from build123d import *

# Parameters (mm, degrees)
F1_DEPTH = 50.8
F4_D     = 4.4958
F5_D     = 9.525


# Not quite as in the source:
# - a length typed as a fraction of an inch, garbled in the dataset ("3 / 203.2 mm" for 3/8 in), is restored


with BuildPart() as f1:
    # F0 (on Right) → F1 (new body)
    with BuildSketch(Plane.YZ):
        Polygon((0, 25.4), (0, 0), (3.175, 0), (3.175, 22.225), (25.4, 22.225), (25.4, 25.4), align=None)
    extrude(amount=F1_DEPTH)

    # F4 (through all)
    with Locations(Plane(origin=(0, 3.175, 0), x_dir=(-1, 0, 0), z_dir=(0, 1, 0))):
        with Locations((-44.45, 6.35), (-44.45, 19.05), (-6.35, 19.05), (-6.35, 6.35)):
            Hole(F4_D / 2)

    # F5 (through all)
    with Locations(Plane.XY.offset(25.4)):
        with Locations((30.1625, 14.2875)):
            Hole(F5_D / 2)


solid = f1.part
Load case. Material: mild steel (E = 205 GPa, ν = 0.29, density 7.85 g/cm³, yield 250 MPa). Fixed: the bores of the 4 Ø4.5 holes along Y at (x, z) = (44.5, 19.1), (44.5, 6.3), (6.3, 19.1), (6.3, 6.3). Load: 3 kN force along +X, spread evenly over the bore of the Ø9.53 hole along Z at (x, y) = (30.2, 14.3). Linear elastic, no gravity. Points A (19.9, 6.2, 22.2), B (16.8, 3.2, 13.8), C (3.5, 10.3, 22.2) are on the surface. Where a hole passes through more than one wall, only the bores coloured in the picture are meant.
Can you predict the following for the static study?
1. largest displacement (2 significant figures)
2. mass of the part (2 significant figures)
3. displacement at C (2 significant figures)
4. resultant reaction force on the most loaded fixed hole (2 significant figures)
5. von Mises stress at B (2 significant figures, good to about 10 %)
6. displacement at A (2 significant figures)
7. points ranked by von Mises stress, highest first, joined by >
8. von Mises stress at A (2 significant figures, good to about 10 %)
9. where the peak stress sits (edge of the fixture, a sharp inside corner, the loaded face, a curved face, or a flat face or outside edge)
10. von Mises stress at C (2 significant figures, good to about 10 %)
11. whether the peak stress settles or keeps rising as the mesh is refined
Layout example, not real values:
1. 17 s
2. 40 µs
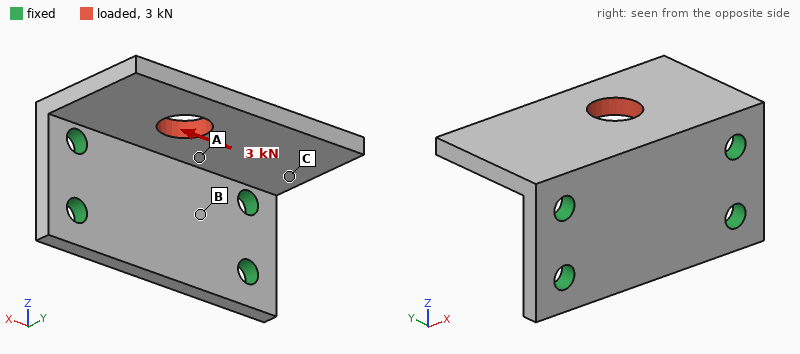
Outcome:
1. 17 µm
2. 57 g
3. 7.8 µm
4. 1.7 kN
5. 13 MPa
6. 3.5 µm
7. A > C > B
8. 44 MPa
9. edge of the fixture
10. 26 MPa
11. keeps rising
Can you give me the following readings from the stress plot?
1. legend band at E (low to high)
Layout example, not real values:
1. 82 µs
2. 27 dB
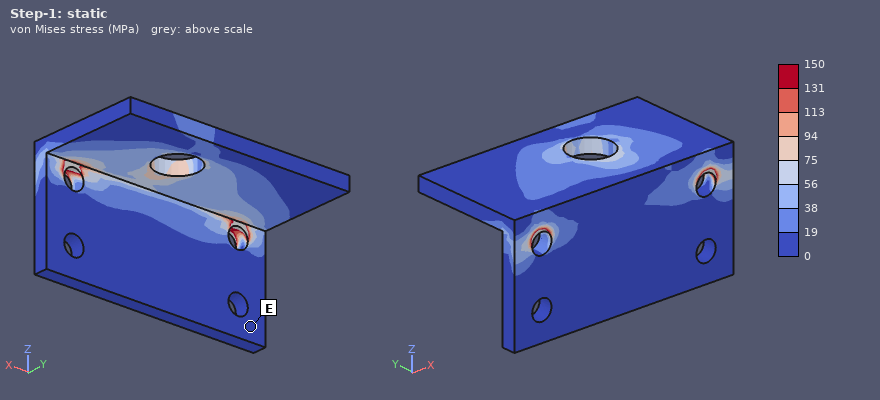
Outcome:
1. 0 to 19 MPa
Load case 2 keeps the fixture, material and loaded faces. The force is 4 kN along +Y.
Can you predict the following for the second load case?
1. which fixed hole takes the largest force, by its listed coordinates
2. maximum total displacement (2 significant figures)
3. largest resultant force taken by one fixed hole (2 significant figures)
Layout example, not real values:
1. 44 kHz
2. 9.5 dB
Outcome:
1. (44.5, 19.1)
2. 49 µm
3. 2.8 kN
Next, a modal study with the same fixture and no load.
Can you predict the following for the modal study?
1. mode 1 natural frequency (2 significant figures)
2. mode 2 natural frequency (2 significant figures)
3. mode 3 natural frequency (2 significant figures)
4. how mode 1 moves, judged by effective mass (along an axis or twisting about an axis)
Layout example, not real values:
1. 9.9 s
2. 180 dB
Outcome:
1. 3600 Hz
2. 5800 Hz
3. 11 kHz
4. along Z
